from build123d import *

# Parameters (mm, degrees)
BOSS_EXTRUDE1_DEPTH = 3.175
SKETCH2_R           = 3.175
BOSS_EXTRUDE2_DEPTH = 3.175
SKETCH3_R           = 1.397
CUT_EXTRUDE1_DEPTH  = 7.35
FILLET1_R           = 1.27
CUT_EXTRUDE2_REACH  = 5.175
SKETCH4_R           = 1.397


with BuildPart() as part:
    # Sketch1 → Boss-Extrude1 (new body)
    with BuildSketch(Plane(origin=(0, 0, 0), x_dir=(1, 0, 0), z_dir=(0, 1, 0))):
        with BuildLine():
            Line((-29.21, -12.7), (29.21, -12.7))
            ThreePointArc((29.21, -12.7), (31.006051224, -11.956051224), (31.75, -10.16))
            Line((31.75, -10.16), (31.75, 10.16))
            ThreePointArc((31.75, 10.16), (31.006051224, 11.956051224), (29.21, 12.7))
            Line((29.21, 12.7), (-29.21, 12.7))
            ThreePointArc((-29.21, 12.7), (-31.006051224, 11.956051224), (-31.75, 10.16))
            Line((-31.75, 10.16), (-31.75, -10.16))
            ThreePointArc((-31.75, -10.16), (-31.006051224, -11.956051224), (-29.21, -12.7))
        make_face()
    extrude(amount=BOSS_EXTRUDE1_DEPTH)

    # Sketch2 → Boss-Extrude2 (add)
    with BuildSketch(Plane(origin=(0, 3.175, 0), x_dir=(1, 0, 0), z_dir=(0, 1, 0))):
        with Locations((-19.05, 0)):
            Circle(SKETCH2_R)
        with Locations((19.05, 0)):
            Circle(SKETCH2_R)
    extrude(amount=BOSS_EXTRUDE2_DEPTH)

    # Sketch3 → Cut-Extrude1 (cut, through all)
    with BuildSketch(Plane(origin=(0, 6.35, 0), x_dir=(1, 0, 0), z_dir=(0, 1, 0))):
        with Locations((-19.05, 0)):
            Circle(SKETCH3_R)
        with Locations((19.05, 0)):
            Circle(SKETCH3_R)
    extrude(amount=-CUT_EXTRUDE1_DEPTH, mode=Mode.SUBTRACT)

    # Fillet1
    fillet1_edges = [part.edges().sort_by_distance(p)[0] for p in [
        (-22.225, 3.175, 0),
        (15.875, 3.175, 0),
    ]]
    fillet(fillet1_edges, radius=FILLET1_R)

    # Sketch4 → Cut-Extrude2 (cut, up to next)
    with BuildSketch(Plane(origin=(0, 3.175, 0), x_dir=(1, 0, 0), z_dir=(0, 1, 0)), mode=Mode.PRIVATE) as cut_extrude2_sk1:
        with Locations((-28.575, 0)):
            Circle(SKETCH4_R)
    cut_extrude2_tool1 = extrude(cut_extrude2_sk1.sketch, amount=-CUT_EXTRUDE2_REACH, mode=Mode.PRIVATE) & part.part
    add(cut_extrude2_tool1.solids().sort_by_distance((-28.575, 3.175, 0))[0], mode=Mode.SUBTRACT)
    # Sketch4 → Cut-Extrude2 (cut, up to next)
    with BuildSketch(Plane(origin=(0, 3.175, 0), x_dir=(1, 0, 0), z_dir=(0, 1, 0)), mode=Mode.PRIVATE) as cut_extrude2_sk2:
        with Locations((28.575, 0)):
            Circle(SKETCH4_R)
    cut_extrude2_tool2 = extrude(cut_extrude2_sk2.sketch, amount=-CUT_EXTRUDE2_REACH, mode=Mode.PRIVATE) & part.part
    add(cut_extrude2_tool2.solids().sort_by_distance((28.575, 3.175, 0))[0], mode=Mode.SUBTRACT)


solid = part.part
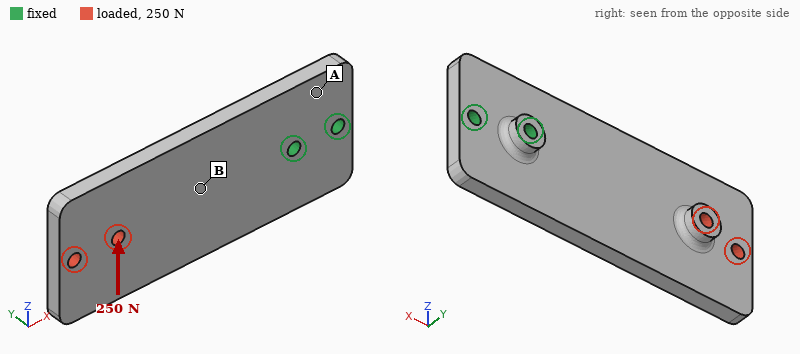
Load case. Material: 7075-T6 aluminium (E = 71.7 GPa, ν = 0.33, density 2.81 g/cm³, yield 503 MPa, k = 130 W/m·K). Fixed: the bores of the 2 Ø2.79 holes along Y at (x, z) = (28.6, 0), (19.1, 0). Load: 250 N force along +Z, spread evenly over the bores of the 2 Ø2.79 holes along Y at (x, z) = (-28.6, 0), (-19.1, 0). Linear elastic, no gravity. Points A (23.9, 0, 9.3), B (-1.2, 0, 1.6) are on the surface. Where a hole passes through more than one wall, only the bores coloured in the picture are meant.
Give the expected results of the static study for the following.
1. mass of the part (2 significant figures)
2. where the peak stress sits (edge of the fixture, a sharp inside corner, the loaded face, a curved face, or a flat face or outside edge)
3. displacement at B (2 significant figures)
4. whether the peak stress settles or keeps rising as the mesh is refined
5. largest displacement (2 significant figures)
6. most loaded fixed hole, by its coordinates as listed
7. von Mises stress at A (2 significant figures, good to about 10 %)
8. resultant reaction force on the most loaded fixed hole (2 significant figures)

15 g
edge of the fixture
22 µm
keeps rising
71 µm
(19.1, 0)
20 MPa
1.0 kN
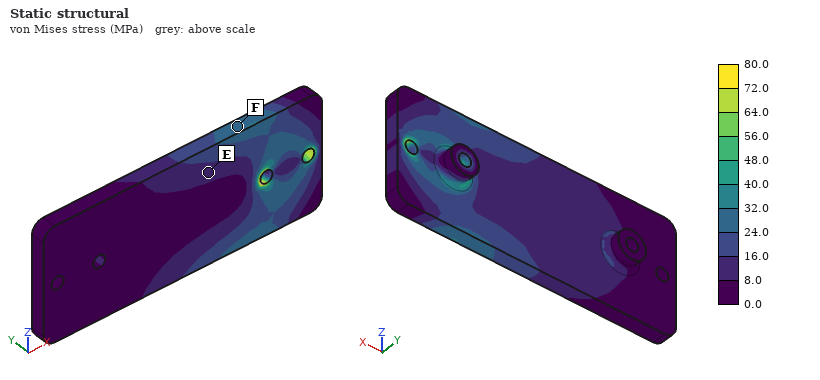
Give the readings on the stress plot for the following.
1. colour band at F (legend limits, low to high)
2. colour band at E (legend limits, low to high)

24.0 to 32.0 MPa
8.0 to 16.0 MPa
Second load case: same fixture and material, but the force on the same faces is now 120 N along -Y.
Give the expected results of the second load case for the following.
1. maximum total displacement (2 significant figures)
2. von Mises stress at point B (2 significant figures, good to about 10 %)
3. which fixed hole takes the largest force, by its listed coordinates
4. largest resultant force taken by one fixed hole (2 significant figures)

0.75 mm
55 MPa
(19.1, 0)
270 N
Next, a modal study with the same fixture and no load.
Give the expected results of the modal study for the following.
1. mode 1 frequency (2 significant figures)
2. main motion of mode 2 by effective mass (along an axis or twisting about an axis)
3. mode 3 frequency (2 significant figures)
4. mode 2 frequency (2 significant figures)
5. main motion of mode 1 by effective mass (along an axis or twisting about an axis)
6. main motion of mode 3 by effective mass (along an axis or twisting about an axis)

1000 Hz
twisting about X
4500 Hz
3800 Hz
along Y
along Z
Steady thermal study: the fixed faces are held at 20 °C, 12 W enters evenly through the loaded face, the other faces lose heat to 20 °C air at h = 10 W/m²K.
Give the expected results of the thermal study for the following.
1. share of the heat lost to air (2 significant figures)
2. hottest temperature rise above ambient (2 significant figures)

7.5 %
50 K
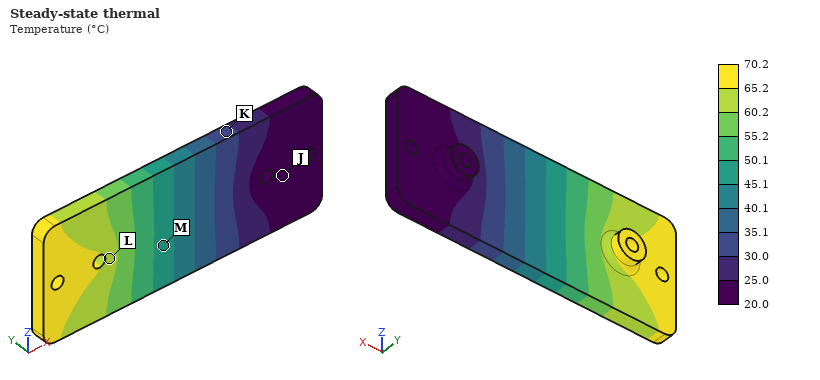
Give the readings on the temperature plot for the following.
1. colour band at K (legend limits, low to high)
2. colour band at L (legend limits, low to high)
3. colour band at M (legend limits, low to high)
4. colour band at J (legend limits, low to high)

30.0 to 35.1 °C
60.2 to 65.2 °C
45.1 to 50.1 °C
20.0 to 25.0 °C
